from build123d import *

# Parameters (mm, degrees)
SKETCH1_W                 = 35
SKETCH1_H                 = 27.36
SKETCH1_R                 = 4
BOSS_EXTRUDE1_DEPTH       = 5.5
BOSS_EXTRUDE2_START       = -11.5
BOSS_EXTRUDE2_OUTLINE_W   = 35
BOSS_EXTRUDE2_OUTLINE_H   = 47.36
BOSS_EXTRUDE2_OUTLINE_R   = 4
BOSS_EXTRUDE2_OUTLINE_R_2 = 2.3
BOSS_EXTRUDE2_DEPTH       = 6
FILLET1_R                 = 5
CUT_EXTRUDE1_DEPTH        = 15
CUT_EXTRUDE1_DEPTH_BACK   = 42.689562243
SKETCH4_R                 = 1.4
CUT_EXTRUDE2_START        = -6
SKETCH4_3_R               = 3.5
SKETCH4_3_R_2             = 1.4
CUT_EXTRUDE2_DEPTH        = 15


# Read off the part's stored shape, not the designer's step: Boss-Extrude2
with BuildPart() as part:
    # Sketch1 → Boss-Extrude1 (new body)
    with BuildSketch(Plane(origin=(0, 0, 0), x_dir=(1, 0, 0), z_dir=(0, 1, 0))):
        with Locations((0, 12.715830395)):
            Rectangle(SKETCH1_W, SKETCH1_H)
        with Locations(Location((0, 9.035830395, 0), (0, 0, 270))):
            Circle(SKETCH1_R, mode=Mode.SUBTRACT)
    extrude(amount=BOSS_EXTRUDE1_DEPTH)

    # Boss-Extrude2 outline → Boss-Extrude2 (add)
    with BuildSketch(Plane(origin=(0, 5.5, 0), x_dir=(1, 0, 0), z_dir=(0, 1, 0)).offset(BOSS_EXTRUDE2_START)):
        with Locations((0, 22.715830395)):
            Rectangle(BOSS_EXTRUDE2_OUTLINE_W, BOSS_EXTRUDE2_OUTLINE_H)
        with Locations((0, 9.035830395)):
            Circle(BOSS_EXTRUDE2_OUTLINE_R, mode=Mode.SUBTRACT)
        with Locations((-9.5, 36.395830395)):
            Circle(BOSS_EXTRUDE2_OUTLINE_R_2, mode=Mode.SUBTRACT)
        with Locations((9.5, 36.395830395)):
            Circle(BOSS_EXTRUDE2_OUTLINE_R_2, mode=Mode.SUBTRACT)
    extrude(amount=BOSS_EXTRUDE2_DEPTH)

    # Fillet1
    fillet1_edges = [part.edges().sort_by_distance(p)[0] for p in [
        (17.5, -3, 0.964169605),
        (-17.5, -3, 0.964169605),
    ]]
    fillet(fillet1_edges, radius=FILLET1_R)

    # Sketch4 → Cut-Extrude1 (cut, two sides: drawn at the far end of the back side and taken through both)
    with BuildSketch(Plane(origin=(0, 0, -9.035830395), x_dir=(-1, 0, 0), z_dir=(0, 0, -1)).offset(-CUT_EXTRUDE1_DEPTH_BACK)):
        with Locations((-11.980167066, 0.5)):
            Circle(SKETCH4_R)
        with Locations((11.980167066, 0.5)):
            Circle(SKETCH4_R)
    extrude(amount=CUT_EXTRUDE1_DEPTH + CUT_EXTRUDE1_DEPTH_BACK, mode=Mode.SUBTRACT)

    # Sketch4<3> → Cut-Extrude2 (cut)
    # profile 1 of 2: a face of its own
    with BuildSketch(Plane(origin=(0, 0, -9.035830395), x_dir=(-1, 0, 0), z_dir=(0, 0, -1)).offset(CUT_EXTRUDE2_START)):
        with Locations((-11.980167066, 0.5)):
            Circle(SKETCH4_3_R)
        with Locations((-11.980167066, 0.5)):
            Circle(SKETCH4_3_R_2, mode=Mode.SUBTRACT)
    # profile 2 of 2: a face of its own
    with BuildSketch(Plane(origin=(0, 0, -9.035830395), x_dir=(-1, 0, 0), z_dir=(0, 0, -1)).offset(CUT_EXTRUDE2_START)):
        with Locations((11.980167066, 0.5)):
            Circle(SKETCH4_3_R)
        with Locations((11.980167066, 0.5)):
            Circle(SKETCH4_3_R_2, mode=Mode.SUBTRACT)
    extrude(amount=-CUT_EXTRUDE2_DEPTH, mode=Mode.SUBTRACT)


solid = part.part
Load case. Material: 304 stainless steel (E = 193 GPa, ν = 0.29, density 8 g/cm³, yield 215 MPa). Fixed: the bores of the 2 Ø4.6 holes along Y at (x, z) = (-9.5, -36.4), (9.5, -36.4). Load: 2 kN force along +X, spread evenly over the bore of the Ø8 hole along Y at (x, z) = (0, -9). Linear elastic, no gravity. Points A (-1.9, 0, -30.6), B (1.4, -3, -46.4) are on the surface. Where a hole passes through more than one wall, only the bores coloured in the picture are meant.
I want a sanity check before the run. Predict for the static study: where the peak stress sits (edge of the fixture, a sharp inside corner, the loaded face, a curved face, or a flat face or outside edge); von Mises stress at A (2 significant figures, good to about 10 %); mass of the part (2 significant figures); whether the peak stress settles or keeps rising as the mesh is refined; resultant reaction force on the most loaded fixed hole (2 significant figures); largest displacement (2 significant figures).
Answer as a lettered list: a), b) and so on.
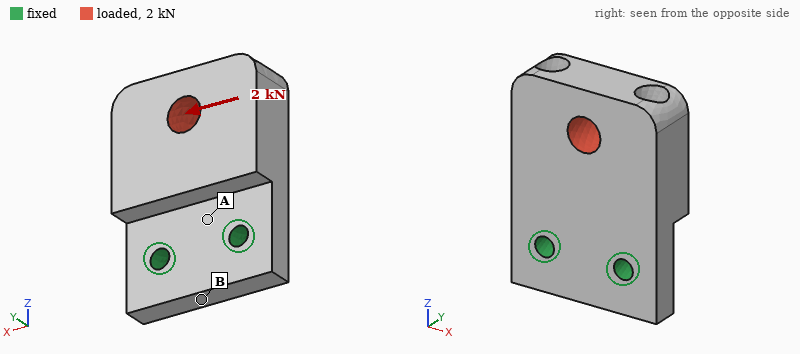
a) edge of the fixture
b) 30 MPa
c) 110 g
d) keeps rising
e) 2.7 kN
f) 11 µm
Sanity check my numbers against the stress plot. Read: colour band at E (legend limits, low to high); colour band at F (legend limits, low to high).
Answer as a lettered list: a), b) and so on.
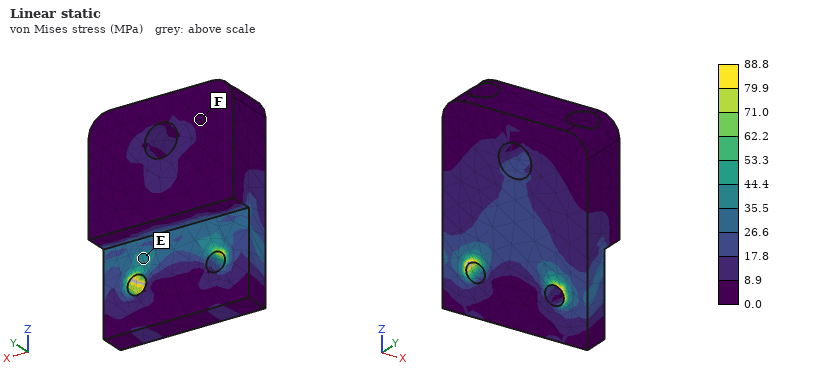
a) 35.5 to 44.4 MPa
b) 0.0 to 8.9 MPa
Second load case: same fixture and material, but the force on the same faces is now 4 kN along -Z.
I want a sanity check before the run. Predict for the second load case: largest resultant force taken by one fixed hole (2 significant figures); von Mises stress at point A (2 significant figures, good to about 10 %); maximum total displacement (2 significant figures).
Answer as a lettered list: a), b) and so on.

a) 2.0 kN
b) 56 MPa
c) 36 µm
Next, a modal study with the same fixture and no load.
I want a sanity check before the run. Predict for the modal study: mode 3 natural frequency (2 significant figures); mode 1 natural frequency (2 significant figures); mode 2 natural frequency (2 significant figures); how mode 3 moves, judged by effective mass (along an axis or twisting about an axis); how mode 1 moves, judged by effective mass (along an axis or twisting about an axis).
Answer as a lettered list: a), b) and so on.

a) 10000 Hz
b) 2900 Hz
c) 9200 Hz
d) along X
e) along Y
